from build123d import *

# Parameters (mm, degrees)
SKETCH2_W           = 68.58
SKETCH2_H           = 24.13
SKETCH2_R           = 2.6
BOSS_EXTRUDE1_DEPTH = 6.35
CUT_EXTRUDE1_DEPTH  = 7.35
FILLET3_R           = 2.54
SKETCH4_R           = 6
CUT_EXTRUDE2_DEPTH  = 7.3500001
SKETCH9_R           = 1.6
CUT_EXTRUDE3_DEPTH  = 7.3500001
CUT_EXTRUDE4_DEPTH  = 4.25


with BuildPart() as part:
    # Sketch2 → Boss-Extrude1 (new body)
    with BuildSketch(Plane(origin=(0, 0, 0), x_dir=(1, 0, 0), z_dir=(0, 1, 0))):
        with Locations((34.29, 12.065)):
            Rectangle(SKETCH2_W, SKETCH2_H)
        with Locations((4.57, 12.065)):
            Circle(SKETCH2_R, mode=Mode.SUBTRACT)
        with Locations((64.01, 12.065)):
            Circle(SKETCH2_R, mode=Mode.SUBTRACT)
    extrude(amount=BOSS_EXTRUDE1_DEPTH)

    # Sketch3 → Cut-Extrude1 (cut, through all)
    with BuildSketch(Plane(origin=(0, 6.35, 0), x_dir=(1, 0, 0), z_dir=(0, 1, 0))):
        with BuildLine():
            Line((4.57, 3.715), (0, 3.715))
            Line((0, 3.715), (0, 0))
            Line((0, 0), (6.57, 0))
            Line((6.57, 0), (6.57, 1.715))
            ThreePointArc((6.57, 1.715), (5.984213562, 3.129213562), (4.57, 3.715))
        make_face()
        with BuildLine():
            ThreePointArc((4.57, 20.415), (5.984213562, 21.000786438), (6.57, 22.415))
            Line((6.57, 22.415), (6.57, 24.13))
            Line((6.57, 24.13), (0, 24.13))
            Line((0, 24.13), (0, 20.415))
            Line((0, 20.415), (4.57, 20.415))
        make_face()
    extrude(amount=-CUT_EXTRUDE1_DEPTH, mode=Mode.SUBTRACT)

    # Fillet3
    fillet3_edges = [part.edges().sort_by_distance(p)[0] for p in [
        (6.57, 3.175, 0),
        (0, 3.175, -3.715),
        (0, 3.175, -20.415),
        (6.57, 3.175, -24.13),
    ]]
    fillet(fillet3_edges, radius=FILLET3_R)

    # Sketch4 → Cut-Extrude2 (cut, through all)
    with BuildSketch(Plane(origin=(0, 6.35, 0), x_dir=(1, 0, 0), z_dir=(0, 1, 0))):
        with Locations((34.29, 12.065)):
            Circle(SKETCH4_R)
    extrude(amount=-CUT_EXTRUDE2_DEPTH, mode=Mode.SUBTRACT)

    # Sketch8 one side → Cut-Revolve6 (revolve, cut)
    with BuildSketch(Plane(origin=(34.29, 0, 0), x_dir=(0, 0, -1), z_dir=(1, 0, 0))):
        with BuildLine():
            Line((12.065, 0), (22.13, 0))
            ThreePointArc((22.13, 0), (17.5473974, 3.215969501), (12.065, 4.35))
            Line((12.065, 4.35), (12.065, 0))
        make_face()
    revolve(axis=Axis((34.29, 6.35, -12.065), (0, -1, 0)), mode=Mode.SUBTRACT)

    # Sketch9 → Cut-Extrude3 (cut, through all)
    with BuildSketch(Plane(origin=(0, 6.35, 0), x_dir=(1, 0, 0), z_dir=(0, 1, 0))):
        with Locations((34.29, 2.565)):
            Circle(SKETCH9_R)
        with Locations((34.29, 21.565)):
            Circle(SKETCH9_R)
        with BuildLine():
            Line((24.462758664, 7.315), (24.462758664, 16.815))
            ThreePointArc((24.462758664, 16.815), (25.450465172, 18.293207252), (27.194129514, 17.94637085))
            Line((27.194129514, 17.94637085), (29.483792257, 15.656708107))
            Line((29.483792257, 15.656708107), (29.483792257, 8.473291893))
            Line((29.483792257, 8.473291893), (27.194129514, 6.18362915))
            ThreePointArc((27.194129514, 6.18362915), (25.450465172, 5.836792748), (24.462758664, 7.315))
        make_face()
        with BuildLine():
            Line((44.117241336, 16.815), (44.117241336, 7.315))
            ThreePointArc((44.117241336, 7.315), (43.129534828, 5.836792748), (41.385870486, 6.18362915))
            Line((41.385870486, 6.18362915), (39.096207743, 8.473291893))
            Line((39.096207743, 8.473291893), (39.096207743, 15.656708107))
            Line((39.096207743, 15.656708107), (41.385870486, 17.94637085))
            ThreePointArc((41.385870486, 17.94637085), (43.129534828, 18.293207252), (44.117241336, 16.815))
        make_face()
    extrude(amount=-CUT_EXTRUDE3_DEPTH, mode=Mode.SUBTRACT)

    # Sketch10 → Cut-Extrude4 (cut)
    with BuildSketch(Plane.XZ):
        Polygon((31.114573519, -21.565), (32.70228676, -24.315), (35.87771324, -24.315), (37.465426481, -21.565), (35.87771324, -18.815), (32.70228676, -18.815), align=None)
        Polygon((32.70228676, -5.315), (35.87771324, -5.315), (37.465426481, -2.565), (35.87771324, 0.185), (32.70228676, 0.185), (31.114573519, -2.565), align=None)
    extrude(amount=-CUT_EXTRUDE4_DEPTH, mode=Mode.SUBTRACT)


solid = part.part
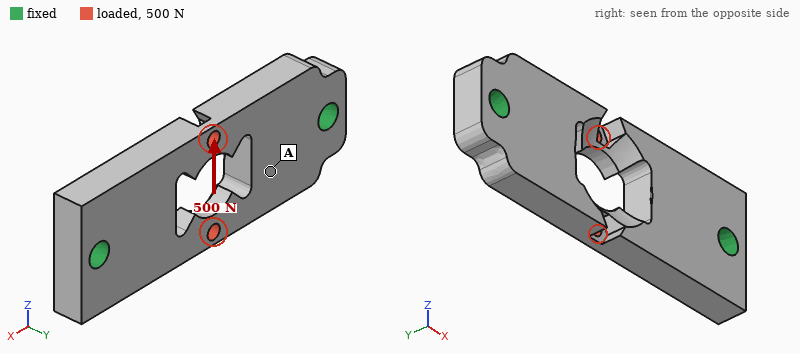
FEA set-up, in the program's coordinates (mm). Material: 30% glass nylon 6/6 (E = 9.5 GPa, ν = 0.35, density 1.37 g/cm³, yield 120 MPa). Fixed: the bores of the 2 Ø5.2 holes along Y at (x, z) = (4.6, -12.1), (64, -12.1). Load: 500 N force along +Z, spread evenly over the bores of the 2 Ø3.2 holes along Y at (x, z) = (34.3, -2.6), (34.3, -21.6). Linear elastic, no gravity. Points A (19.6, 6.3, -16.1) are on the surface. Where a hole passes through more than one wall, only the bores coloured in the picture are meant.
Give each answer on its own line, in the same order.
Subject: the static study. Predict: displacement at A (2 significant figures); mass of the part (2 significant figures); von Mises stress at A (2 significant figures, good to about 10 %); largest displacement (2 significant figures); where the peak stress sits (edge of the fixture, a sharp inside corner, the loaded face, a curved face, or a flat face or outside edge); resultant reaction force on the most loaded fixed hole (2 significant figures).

0.044 mm
11 g
12 MPa
0.14 mm
the loaded face
250 N
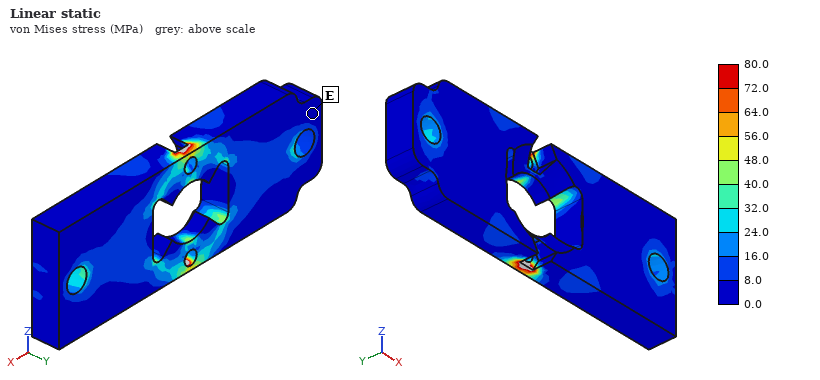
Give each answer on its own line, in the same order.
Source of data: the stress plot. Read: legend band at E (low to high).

0.0 to 8.0 MPa
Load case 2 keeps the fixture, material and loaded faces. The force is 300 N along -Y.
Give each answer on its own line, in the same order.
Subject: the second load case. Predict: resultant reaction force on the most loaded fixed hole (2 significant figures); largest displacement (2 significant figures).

330 N
0.20 mm
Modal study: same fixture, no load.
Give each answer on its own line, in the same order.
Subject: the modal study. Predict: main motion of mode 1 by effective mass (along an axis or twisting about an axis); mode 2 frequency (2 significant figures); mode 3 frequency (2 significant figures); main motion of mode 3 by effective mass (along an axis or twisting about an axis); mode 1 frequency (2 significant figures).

along Y
6100 Hz
7600 Hz
along Z
4500 Hz
